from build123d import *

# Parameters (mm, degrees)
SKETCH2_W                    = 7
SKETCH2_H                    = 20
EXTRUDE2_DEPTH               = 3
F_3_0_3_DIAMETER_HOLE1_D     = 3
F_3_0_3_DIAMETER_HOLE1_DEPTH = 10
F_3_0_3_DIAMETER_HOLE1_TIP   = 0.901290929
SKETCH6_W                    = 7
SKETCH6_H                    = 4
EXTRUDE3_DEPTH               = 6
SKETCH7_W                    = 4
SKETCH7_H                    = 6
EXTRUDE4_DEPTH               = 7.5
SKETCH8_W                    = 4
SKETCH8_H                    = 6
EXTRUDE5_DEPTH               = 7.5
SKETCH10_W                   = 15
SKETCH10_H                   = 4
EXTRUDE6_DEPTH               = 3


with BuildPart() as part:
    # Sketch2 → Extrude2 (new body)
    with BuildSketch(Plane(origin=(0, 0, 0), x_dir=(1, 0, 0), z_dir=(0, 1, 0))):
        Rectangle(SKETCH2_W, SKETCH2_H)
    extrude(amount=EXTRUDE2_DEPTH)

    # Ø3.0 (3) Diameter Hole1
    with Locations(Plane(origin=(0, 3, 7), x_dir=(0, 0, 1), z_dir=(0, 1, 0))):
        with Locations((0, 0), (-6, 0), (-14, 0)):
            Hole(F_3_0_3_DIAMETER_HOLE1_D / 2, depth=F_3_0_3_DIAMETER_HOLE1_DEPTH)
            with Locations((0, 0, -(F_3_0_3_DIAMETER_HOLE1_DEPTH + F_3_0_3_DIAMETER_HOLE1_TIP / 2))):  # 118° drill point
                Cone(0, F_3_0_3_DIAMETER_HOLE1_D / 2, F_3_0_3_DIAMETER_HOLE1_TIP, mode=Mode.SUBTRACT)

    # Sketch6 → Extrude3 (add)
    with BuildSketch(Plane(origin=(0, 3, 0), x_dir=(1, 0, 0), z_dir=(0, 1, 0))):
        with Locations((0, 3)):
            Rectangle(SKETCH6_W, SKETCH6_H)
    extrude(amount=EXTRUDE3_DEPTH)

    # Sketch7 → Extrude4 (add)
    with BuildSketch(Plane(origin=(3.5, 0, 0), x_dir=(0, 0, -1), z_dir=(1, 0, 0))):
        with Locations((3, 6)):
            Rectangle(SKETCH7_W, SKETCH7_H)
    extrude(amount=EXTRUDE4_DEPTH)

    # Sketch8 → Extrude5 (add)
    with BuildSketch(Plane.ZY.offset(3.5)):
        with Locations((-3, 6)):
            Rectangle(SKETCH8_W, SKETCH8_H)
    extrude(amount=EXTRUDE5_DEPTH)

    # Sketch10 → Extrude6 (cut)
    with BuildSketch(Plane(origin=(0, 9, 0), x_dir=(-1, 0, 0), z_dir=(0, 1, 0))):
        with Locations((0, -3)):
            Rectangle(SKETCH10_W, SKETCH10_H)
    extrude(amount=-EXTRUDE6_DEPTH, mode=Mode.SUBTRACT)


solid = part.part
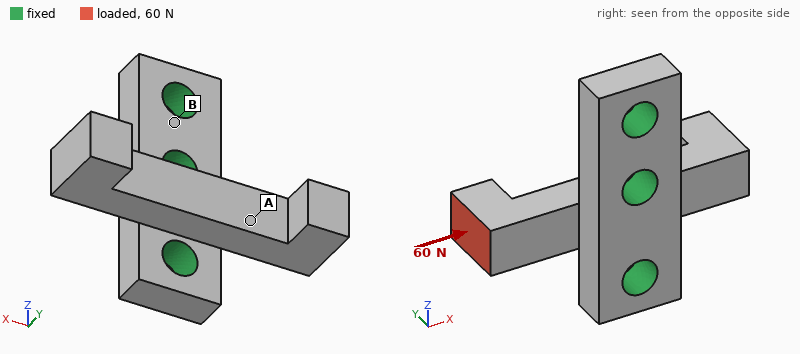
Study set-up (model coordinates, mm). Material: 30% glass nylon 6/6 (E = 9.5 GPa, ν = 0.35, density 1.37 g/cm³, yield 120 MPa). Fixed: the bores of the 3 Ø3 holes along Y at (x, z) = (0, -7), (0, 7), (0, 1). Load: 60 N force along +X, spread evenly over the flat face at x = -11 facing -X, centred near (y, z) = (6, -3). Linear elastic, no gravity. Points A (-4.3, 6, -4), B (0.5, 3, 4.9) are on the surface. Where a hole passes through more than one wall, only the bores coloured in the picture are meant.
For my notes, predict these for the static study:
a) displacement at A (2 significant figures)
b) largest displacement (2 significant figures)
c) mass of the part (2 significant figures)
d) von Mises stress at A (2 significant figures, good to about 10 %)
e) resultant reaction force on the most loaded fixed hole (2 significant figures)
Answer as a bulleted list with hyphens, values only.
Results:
- 18 µm
- 82 µm
- 0.97 g
- 20 MPa
- 33 N
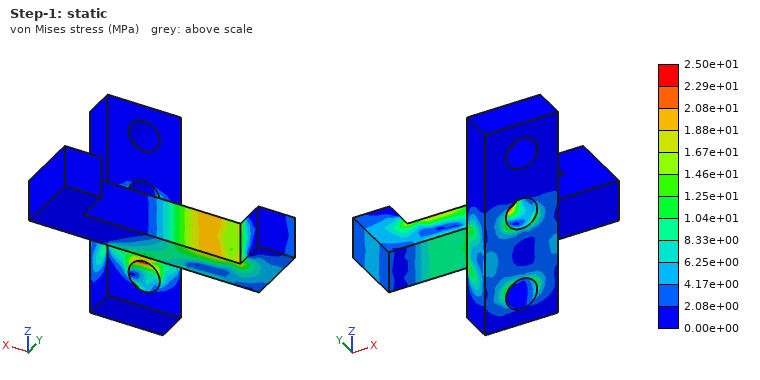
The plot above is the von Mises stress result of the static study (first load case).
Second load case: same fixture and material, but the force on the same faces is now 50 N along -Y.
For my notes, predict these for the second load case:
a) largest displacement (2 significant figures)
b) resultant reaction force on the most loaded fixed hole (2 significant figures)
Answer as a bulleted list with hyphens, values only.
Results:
- 0.22 mm
- 37 N
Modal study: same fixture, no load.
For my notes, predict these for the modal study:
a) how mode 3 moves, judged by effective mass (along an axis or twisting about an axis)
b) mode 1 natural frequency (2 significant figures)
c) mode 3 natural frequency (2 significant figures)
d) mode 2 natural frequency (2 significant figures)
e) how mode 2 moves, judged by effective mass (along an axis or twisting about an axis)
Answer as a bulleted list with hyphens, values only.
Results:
- twisting about Y
- 7900 Hz
- 10 kHz
- 10000 Hz
- along Y
